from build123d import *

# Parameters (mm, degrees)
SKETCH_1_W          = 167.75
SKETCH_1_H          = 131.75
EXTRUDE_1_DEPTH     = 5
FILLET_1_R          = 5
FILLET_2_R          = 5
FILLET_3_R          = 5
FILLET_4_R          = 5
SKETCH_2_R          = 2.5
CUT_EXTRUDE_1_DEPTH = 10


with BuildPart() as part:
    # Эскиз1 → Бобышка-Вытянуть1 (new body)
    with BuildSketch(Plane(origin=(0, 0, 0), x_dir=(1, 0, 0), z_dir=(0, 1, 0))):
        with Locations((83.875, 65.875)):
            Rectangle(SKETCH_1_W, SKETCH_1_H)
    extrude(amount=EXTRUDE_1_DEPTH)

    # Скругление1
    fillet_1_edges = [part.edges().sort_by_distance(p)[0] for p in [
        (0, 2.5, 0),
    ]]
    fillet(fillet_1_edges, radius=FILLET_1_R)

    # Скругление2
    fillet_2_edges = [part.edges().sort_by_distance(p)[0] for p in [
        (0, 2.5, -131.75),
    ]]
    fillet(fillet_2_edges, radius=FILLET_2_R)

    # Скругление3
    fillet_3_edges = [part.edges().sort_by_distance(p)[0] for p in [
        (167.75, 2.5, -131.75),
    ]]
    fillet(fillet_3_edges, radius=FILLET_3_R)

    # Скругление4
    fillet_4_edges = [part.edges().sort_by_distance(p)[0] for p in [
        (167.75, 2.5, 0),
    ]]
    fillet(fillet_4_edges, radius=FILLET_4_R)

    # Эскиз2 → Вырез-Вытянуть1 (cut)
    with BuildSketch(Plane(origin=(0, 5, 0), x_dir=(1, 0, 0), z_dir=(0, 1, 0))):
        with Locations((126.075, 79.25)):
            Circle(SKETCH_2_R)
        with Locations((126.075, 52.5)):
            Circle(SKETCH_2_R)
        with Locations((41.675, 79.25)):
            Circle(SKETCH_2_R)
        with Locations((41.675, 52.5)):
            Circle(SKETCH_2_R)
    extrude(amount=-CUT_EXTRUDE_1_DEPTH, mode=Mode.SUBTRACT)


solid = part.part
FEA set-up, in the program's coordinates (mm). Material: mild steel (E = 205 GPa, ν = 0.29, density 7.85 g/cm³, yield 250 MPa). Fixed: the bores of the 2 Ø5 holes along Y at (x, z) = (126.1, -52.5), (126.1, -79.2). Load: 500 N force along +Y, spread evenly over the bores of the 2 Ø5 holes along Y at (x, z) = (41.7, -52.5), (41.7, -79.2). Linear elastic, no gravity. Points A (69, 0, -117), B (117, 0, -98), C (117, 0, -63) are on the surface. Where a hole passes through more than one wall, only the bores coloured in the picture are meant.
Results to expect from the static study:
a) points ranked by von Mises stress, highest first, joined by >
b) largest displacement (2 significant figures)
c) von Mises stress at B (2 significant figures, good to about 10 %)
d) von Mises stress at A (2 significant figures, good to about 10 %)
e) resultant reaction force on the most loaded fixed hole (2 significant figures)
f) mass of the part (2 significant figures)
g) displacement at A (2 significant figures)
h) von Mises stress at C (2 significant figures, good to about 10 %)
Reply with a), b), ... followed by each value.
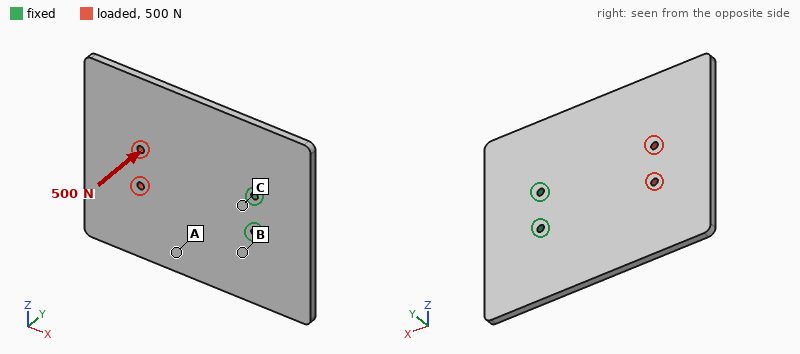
a) C > B > A
b) 0.78 mm
c) 59 MPa
d) 25 MPa
e) 250 N
f) 860 g
g) 0.26 mm
h) 91 MPa
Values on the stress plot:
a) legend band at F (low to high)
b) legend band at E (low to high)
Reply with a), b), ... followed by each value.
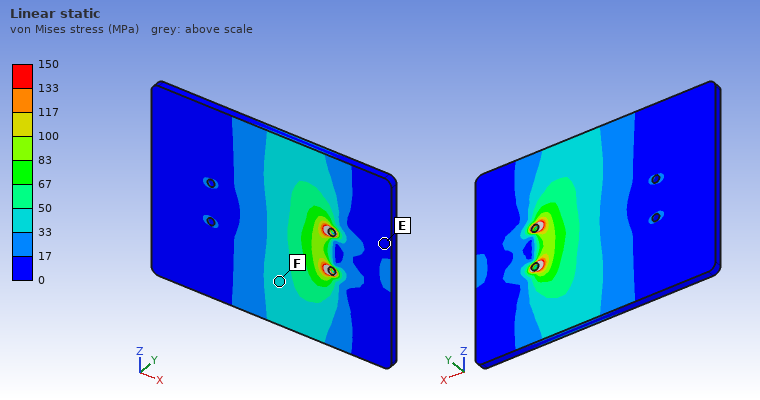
a) 33 to 50 MPa
b) 0 to 17 MPa
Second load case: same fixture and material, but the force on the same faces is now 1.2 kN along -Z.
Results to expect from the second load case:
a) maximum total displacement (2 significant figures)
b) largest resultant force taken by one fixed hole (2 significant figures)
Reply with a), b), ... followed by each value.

a) 29 µm
b) 3.5 kN
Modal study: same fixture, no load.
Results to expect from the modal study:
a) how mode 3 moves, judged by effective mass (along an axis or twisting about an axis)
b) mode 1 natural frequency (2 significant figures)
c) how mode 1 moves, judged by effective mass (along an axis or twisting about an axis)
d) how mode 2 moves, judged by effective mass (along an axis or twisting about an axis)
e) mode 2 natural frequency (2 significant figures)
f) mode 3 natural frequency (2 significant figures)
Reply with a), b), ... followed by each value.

a) along Y
b) 230 Hz
c) along Y
d) twisting about X
e) 500 Hz
f) 1200 Hz
